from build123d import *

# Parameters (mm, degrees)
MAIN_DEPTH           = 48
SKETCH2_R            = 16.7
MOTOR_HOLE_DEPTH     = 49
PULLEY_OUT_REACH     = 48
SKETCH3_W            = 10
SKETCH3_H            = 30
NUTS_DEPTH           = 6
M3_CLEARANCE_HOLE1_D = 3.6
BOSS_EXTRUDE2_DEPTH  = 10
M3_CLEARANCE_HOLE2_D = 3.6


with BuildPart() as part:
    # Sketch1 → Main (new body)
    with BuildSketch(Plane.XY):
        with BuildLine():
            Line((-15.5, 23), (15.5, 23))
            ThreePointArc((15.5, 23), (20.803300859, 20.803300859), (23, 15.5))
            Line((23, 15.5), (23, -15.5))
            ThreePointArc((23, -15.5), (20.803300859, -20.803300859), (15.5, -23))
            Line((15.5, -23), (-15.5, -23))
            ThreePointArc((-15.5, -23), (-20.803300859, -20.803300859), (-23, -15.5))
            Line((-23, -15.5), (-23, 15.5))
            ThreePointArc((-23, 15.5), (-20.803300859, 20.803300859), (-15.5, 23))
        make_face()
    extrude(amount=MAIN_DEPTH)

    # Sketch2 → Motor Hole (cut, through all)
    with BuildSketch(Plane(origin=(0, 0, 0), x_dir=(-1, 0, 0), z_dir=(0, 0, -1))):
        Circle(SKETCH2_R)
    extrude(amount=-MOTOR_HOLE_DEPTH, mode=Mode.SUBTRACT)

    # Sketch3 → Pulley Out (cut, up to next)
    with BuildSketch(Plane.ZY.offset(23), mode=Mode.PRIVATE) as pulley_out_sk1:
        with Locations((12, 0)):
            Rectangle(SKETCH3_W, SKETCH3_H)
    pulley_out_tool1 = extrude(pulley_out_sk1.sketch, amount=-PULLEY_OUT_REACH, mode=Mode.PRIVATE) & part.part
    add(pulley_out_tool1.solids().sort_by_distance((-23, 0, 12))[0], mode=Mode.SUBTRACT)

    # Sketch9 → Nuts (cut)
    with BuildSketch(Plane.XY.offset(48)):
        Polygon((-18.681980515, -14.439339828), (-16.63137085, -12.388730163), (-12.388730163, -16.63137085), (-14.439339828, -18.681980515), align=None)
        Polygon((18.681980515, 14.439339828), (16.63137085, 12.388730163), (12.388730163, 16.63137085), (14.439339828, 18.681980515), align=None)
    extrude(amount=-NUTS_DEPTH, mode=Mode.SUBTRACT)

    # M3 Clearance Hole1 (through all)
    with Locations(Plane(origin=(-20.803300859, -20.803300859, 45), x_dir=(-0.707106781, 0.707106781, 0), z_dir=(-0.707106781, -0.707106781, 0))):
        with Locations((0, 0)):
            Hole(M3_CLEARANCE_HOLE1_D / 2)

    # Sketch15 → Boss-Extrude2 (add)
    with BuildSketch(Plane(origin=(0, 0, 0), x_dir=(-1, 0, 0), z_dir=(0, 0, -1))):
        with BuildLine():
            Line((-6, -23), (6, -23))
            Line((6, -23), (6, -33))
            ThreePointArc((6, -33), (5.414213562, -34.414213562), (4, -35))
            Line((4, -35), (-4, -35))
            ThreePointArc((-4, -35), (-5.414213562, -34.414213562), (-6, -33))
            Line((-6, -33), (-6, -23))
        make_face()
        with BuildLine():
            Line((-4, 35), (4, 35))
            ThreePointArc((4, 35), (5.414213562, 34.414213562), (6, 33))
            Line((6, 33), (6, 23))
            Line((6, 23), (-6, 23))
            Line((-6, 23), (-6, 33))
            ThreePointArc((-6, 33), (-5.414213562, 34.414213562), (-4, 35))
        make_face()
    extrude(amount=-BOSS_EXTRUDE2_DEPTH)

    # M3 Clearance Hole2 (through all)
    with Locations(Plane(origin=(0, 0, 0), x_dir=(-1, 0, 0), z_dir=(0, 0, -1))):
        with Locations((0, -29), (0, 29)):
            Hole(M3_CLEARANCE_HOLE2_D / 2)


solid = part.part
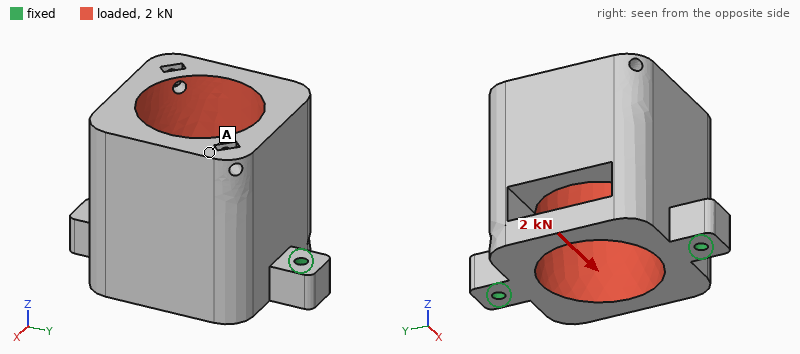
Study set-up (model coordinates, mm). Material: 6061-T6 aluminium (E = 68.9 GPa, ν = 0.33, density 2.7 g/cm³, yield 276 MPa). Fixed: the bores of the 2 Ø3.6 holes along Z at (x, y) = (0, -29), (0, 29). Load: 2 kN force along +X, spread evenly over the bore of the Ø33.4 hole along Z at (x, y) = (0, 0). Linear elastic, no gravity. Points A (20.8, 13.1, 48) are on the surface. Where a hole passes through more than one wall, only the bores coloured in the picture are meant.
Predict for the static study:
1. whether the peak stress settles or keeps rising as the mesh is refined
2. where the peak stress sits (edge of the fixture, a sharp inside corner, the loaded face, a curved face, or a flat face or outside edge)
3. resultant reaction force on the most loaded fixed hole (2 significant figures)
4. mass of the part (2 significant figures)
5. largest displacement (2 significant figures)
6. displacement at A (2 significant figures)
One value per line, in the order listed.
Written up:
keeps rising
edge of the fixture
1.0 kN
150 g
0.16 mm
0.15 mm
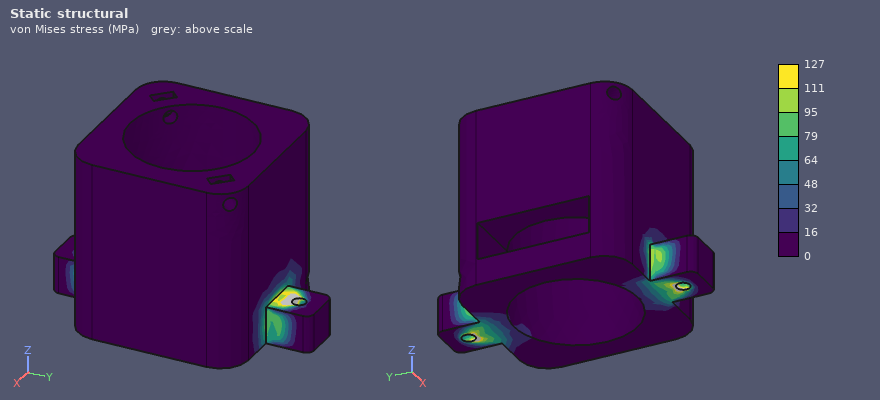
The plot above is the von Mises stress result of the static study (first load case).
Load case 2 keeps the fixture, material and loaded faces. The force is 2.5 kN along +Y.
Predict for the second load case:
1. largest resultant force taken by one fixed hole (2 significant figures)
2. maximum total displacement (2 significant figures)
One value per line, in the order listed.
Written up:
1.6 kN
16 µm
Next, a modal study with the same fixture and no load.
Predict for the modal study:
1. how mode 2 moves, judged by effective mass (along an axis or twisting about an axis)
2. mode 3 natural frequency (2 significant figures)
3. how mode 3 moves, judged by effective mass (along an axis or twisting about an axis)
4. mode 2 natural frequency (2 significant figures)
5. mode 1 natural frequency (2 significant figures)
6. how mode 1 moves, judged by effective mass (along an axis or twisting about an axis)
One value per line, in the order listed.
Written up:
along Y
7500 Hz
along Z
6000 Hz
1600 Hz
along X
